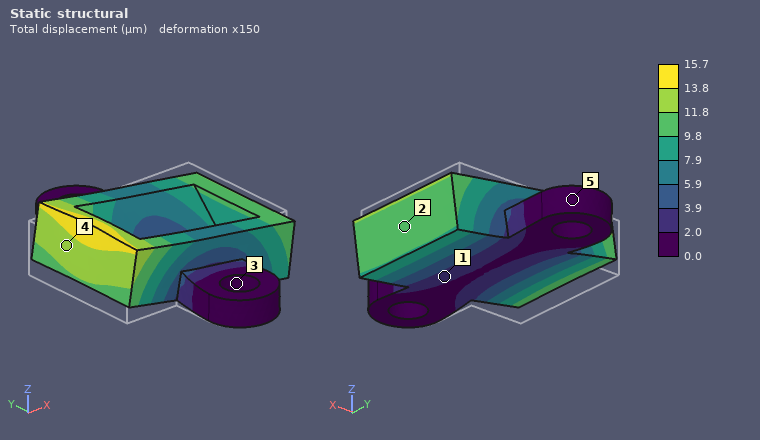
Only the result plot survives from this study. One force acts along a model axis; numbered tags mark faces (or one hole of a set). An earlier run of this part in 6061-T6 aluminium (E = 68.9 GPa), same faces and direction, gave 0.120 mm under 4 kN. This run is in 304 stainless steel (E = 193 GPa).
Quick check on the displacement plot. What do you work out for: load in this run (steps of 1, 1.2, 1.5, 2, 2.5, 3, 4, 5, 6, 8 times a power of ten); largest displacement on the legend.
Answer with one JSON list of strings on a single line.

["1.5 kN", "15.7 µm"]
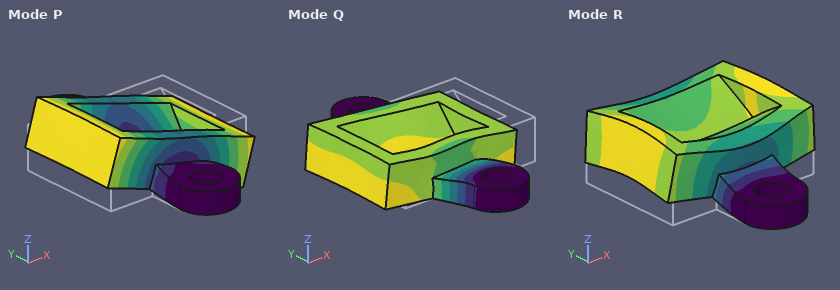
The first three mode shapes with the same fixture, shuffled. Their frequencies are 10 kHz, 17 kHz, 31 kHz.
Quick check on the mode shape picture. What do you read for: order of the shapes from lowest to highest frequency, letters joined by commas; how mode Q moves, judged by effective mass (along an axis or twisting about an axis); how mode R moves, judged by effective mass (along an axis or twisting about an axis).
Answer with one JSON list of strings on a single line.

["P, R, Q", "along X", "along Z"]
